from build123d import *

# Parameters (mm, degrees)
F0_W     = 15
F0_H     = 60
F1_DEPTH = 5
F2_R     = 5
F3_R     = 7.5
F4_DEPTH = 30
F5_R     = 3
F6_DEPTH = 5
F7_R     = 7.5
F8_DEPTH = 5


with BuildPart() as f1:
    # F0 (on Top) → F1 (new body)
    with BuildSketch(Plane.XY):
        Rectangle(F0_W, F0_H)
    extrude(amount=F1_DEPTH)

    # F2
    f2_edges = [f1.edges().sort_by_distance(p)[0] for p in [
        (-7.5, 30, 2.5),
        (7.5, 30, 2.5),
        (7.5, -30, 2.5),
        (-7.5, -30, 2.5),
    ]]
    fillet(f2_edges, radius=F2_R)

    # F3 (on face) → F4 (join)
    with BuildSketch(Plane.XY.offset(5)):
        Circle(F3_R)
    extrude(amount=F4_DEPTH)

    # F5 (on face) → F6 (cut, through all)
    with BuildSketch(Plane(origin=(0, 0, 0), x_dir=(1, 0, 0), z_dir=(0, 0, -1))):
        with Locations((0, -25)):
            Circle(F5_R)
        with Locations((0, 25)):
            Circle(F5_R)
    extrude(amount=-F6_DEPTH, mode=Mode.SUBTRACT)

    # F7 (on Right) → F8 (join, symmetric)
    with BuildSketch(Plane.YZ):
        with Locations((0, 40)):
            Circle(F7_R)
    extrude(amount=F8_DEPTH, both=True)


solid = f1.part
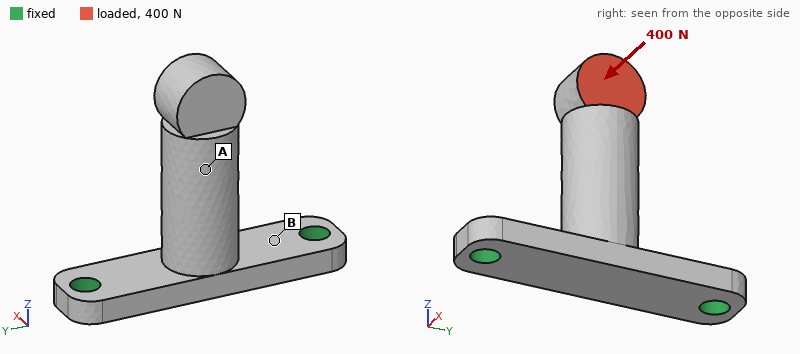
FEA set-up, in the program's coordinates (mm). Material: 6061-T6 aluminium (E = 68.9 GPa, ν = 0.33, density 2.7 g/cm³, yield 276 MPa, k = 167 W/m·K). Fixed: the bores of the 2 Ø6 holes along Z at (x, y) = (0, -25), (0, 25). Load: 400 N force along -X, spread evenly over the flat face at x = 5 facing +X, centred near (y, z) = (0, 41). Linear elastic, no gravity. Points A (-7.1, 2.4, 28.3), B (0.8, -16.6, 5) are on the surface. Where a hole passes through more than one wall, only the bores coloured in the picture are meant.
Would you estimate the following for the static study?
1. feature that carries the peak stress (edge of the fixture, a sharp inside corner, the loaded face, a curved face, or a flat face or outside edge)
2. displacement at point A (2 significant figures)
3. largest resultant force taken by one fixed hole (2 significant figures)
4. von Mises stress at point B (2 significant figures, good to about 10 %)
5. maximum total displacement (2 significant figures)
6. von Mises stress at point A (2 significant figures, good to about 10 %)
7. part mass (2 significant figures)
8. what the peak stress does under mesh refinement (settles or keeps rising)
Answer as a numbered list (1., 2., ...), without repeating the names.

1. edge of the fixture
2. 0.28 mm
3. 200 N
4. 120 MPa
5. 0.49 mm
6. 14 MPa
7. 30 g
8. keeps rising
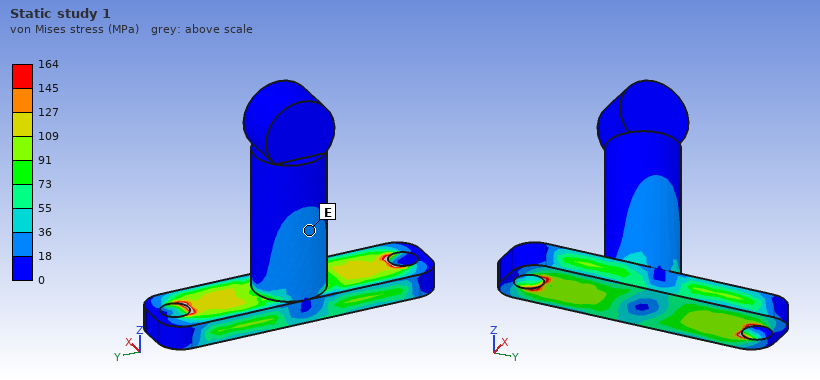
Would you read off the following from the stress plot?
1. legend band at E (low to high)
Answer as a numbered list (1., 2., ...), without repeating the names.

1. 18 to 36 MPa
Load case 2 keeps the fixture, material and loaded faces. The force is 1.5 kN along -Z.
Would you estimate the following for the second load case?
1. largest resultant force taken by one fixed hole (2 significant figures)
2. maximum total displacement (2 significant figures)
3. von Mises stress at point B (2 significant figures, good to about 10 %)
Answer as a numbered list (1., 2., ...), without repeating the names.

1. 790 N
2. 0.27 mm
3. 62 MPa
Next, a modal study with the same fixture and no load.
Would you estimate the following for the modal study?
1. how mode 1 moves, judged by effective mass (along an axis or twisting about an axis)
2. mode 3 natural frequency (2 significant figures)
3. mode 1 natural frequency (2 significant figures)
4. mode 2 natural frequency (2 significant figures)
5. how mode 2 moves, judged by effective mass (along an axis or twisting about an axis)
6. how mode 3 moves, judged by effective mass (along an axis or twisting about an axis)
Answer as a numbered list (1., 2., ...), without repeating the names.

1. along X
2. 5800 Hz
3. 1700 Hz
4. 3400 Hz
5. along Y
6. along Z
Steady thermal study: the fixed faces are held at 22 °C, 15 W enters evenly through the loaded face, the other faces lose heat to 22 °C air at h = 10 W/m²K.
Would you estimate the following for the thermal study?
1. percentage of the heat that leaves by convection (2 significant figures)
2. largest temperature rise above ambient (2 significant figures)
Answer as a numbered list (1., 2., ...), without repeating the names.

1. 3.6 %
2. 33 K
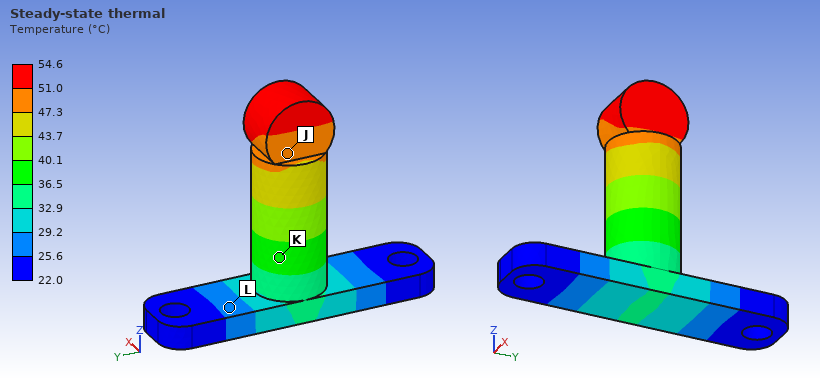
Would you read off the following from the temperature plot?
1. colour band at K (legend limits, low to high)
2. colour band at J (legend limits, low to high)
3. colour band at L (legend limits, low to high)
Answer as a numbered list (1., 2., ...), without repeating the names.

1. 36.5 to 40.1 °C
2. 47.3 to 51.0 °C
3. 25.6 to 29.2 °C
